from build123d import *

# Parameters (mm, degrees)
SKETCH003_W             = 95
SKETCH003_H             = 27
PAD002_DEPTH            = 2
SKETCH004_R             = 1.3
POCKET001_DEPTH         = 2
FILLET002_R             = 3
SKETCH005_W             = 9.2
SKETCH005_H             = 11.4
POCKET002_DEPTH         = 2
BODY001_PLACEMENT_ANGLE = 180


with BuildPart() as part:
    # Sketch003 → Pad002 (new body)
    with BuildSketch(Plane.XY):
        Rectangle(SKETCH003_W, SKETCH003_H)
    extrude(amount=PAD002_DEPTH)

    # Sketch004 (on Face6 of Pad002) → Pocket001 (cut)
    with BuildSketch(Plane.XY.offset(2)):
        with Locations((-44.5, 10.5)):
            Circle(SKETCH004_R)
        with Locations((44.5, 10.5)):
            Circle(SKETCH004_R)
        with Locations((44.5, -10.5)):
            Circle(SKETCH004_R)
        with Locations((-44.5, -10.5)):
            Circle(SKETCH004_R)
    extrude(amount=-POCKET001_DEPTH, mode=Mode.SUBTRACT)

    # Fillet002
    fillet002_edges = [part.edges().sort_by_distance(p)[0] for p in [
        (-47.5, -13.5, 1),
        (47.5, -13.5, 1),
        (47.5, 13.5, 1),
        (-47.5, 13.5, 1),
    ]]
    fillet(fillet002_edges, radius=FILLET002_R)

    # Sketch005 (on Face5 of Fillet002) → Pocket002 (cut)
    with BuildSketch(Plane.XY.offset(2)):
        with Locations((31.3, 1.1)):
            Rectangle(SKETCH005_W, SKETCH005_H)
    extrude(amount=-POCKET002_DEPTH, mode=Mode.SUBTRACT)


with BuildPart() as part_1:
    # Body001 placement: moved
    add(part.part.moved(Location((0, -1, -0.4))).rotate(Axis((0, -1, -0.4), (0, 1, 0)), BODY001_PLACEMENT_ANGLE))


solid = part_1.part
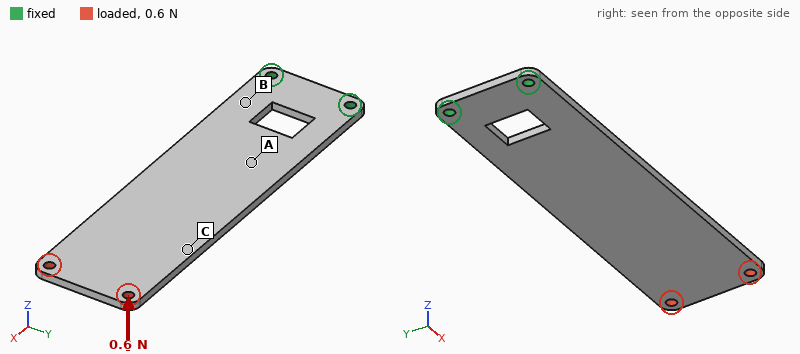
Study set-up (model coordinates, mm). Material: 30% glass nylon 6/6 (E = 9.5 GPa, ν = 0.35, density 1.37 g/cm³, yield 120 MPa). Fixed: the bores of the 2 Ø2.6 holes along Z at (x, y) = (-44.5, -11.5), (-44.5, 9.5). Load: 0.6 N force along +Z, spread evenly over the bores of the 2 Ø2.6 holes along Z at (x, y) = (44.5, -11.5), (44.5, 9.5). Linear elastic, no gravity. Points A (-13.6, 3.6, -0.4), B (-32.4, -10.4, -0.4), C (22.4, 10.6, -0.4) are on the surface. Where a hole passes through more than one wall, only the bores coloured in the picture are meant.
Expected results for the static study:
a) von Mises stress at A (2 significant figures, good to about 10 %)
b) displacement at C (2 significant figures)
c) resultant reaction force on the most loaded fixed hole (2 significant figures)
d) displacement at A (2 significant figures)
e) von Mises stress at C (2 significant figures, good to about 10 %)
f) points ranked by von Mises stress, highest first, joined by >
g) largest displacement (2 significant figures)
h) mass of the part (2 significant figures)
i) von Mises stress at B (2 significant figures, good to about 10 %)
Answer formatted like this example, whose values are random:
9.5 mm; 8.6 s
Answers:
1.9 MPa; 0.69 mm; 0.32 N; 0.19 mm; 0.75 MPa; B > A > C; 1.1 mm; 6.7 g; 4.3 MPa
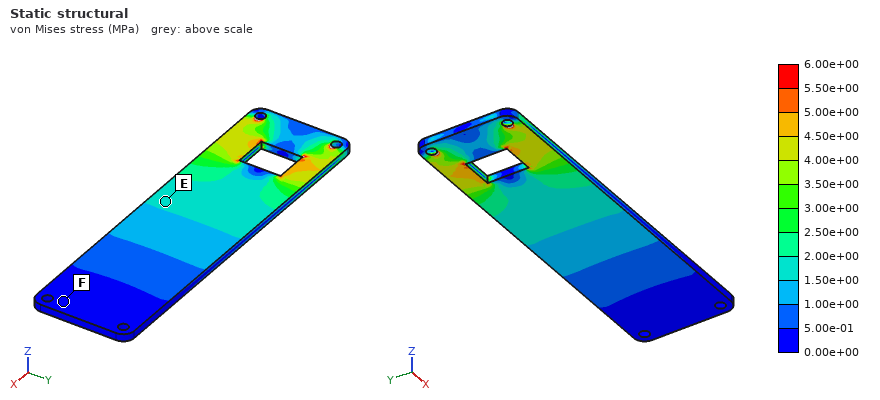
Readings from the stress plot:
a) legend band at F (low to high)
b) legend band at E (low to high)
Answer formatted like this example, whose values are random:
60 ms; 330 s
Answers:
0.00e+00 to 5.00e-01 MPa; 1.50e+00 to 2.00e+00 MPa
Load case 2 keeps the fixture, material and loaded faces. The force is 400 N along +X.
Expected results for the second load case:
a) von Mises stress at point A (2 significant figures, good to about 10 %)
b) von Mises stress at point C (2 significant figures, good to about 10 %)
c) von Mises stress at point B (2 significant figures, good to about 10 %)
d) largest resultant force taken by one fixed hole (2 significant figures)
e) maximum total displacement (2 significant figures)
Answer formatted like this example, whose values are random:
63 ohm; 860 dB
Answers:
6.3 MPa; 7.6 MPa; 12 MPa; 200 N; 0.10 mm
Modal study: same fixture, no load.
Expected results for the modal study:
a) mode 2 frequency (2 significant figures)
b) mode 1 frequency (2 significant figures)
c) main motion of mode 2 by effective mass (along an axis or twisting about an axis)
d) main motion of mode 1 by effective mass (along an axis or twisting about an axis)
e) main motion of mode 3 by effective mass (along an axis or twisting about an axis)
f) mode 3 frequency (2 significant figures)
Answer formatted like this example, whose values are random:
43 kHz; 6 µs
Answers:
620 Hz; 88 Hz; along Z; along Z; twisting about X; 660 Hz
